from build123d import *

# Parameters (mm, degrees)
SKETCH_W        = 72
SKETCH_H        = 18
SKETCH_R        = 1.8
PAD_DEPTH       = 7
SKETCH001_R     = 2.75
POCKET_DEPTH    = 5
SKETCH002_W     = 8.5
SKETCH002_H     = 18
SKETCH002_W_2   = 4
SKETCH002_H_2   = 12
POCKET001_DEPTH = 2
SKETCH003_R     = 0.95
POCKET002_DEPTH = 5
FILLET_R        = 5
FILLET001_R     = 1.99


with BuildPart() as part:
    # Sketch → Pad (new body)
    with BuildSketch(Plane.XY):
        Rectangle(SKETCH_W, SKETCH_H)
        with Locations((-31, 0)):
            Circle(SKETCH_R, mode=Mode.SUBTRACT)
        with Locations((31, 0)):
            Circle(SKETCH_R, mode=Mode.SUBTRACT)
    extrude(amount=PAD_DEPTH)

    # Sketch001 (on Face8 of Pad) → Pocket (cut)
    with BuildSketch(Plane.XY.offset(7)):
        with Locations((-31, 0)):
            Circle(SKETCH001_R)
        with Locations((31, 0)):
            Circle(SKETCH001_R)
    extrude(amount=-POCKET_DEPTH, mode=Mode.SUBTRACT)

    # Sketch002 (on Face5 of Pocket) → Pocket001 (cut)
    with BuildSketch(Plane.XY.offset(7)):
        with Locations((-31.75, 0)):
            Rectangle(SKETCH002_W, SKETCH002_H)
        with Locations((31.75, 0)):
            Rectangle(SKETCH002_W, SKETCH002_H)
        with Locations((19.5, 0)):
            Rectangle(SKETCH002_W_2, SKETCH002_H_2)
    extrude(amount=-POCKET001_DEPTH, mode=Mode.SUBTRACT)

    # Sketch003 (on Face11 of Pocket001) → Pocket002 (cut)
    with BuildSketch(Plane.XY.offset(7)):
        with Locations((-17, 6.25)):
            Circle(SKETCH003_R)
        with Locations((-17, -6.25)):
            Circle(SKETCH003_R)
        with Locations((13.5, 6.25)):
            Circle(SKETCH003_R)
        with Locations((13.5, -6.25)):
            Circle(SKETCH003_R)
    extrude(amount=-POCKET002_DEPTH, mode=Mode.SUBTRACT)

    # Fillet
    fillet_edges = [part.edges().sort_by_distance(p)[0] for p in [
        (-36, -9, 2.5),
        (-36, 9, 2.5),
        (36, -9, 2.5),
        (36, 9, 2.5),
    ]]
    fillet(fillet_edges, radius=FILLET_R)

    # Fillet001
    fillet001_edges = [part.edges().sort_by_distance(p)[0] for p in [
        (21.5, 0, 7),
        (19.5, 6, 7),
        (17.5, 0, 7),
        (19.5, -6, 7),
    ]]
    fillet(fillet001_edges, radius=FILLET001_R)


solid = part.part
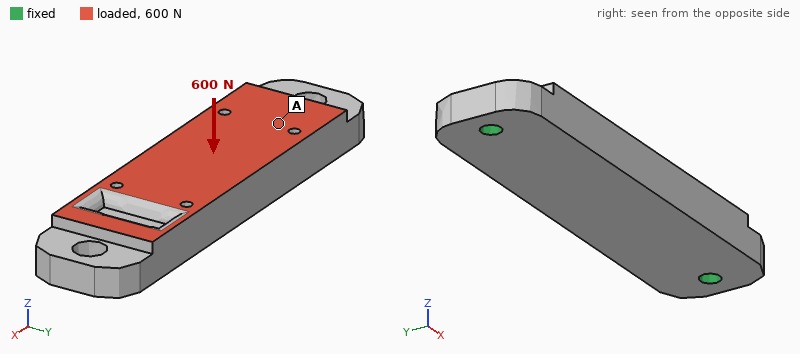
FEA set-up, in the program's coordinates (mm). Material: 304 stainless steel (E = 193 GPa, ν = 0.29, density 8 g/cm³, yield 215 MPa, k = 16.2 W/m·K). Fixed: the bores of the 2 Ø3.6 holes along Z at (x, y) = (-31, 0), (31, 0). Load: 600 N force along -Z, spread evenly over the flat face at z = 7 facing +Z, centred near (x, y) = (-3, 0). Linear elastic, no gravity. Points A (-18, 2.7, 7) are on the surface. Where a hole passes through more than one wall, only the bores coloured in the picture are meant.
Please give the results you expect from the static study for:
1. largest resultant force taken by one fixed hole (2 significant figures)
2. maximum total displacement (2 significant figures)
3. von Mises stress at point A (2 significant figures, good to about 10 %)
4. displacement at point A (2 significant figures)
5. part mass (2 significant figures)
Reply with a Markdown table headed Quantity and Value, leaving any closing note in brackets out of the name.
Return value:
| Quantity | Value |
|---|---|
| largest resultant force taken by one fixed hole | 600 N |
| maximum total displacement | 11 µm |
| von Mises stress at point A | 13 MPa |
| displacement at point A | 6.4 µm |
| part mass | 64 g |
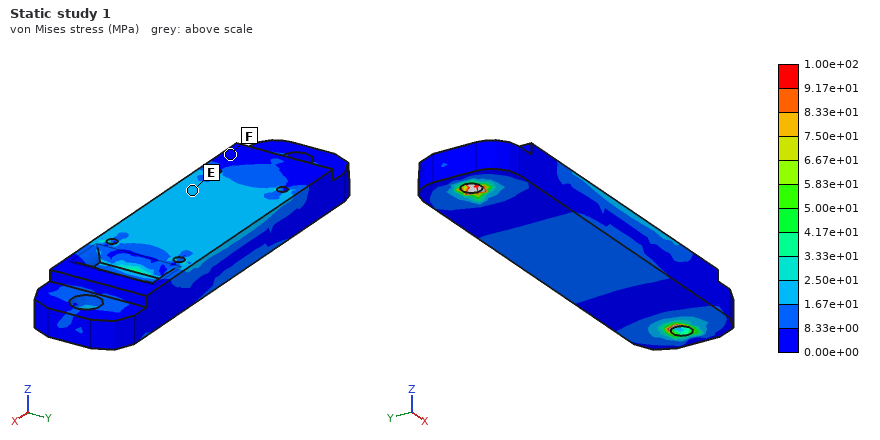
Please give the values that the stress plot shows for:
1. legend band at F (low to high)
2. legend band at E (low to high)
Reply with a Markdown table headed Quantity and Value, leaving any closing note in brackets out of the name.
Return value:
| Quantity | Value |
|---|---|
| legend band at F | 0.00e+00 to 8.33e+00 MPa |
| legend band at E | 1.67e+01 to 2.50e+01 MPa |
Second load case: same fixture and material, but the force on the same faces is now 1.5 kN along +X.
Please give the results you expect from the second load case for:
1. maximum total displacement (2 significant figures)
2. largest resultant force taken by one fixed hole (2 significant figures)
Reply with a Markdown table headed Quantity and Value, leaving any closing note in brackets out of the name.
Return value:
| Quantity | Value |
|---|---|
| maximum total displacement | 2.0 µm |
| largest resultant force taken by one fixed hole | 770 N |
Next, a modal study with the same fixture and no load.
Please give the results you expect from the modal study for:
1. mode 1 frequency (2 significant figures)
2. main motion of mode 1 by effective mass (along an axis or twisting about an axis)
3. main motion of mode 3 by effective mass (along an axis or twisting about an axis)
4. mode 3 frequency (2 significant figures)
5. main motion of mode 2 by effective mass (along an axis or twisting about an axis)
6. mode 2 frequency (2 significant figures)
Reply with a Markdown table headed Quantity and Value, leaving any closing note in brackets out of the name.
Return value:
| Quantity | Value |
|---|---|
| mode 1 frequency | 5800 Hz |
| main motion of mode 1 by effective mass | along Z |
| main motion of mode 3 by effective mass | along Y |
| mode 3 frequency | 11 kHz |
| main motion of mode 2 by effective mass | along Y |
| mode 2 frequency | 7100 Hz |
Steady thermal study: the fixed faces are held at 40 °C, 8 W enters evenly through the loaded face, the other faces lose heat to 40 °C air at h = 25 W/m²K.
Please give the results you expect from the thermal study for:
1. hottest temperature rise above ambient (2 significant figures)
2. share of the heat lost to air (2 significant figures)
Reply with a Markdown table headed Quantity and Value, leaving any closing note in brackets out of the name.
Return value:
| Quantity | Value |
|---|---|
| hottest temperature rise above ambient | 44 K |
| share of the heat lost to air | 25 % |
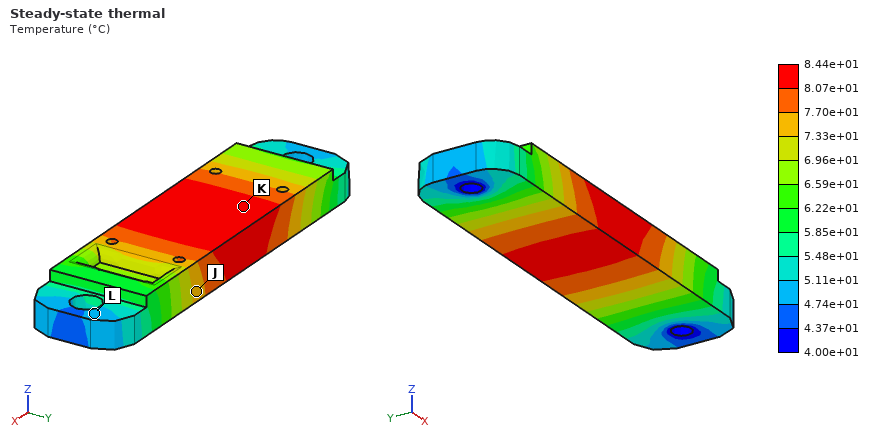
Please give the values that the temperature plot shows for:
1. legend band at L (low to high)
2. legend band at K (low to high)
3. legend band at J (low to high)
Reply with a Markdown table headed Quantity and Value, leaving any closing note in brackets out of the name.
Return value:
| Quantity | Value |
|---|---|
| legend band at L | 4.74e+01 to 5.11e+01 °C |
| legend band at K | 8.07e+01 to 8.44e+01 °C |
| legend band at J | 7.33e+01 to 7.70e+01 °C |
